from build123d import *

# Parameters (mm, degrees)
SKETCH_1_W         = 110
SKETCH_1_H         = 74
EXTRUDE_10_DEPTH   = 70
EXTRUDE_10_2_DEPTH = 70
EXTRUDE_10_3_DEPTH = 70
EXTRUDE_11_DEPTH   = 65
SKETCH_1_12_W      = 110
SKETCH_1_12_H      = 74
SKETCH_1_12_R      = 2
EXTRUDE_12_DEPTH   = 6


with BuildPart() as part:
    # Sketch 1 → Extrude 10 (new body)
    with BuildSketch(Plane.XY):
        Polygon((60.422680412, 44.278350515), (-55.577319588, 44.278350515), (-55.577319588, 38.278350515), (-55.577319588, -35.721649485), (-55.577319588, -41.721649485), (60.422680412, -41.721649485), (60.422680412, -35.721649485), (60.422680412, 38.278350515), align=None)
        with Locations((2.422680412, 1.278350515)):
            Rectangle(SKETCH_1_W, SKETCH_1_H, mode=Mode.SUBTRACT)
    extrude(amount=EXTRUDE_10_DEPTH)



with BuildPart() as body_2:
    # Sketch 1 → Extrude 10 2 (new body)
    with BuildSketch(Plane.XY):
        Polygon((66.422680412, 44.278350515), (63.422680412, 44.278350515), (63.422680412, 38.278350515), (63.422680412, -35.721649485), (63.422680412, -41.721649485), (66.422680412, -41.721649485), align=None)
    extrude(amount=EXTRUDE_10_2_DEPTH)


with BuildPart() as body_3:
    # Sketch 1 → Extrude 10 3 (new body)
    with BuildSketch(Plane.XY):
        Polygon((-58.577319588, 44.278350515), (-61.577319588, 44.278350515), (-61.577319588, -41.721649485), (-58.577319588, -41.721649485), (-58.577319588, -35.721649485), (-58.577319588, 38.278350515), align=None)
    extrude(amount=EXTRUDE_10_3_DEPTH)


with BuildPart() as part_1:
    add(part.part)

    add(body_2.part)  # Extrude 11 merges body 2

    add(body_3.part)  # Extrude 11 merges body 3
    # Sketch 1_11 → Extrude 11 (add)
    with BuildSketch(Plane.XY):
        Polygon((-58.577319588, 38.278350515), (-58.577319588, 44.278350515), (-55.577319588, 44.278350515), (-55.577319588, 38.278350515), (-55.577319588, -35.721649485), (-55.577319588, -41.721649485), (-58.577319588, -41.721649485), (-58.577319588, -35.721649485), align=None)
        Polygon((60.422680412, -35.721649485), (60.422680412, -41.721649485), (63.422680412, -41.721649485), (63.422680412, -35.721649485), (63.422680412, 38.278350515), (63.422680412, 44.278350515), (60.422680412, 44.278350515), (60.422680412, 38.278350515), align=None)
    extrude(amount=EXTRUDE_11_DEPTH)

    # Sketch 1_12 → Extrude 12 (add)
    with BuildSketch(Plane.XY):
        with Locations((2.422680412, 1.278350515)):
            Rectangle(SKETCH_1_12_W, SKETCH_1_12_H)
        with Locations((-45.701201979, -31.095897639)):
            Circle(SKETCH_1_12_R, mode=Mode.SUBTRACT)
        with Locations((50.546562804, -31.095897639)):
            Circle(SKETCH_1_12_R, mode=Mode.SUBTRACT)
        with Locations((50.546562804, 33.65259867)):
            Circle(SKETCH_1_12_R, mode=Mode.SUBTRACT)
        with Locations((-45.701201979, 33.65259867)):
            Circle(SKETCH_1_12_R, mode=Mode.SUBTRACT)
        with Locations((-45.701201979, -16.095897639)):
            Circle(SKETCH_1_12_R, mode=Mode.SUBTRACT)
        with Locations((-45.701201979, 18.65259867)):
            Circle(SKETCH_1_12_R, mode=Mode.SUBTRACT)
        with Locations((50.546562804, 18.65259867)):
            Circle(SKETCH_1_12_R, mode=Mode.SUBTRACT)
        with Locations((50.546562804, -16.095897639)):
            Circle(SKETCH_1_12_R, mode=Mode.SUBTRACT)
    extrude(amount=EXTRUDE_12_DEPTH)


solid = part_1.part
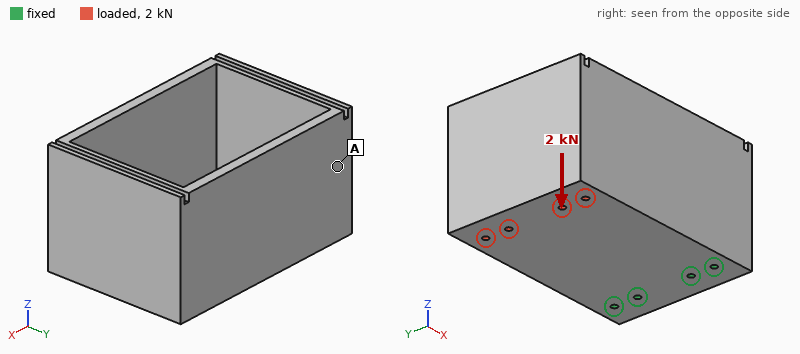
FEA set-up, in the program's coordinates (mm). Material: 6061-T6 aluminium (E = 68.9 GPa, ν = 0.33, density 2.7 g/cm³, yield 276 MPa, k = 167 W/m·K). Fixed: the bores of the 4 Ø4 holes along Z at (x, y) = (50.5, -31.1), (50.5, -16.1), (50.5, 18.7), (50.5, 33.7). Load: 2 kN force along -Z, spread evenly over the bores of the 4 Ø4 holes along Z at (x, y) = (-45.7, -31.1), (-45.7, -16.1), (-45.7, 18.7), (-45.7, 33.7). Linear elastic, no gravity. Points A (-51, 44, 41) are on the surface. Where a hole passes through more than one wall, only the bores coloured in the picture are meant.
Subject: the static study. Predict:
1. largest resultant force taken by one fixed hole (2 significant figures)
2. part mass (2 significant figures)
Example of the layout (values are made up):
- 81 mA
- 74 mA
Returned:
- 2.1 kN
- 670 g
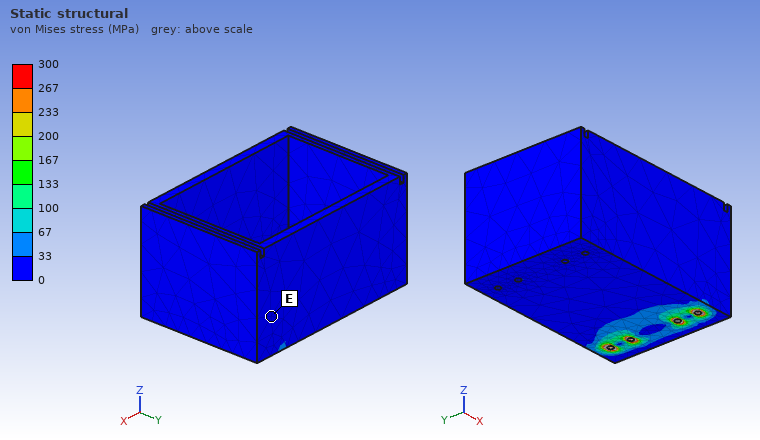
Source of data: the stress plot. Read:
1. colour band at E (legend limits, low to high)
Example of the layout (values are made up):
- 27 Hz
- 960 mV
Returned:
- 0 to 33 MPa
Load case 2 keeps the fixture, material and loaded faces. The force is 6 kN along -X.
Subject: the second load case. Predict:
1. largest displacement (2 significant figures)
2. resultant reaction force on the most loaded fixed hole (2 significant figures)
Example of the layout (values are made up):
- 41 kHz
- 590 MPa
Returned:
- 22 µm
- 1.7 kN
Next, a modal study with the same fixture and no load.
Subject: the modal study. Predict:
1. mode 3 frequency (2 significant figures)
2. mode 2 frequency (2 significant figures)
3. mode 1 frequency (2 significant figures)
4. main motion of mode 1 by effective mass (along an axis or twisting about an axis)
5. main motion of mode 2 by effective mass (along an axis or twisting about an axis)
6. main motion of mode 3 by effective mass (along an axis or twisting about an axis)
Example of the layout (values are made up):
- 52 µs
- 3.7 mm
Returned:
- 2100 Hz
- 860 Hz
- 390 Hz
- along Z
- along Y
- along Y
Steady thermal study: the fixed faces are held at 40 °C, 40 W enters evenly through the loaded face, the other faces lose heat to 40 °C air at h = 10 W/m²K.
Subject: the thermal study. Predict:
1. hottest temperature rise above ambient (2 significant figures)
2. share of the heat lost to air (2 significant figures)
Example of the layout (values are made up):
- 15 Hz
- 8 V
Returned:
- 23 K
- 20 %
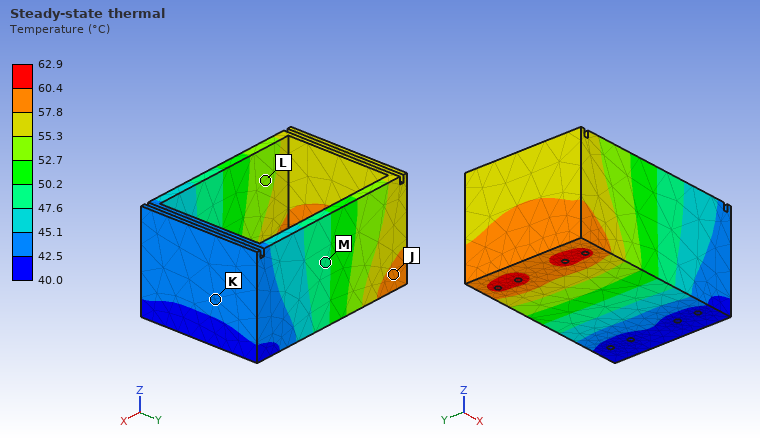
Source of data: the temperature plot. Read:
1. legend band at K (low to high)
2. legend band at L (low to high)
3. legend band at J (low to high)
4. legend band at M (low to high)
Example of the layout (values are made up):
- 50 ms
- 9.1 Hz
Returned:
- 42.5 to 45.1 °C
- 52.7 to 55.3 °C
- 57.8 to 60.4 °C
- 47.6 to 50.2 °C
